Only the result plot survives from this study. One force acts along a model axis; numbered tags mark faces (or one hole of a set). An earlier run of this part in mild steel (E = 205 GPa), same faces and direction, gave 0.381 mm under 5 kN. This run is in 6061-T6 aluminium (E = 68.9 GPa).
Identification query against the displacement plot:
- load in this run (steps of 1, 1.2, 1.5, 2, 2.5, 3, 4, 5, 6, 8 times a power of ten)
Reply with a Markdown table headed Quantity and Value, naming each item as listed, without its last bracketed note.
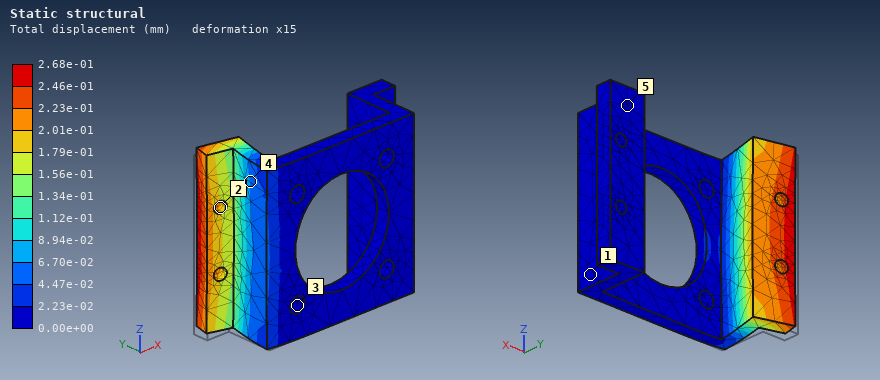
| Quantity | Value |
|---|---|
| load in this run | 1.2 kN |
